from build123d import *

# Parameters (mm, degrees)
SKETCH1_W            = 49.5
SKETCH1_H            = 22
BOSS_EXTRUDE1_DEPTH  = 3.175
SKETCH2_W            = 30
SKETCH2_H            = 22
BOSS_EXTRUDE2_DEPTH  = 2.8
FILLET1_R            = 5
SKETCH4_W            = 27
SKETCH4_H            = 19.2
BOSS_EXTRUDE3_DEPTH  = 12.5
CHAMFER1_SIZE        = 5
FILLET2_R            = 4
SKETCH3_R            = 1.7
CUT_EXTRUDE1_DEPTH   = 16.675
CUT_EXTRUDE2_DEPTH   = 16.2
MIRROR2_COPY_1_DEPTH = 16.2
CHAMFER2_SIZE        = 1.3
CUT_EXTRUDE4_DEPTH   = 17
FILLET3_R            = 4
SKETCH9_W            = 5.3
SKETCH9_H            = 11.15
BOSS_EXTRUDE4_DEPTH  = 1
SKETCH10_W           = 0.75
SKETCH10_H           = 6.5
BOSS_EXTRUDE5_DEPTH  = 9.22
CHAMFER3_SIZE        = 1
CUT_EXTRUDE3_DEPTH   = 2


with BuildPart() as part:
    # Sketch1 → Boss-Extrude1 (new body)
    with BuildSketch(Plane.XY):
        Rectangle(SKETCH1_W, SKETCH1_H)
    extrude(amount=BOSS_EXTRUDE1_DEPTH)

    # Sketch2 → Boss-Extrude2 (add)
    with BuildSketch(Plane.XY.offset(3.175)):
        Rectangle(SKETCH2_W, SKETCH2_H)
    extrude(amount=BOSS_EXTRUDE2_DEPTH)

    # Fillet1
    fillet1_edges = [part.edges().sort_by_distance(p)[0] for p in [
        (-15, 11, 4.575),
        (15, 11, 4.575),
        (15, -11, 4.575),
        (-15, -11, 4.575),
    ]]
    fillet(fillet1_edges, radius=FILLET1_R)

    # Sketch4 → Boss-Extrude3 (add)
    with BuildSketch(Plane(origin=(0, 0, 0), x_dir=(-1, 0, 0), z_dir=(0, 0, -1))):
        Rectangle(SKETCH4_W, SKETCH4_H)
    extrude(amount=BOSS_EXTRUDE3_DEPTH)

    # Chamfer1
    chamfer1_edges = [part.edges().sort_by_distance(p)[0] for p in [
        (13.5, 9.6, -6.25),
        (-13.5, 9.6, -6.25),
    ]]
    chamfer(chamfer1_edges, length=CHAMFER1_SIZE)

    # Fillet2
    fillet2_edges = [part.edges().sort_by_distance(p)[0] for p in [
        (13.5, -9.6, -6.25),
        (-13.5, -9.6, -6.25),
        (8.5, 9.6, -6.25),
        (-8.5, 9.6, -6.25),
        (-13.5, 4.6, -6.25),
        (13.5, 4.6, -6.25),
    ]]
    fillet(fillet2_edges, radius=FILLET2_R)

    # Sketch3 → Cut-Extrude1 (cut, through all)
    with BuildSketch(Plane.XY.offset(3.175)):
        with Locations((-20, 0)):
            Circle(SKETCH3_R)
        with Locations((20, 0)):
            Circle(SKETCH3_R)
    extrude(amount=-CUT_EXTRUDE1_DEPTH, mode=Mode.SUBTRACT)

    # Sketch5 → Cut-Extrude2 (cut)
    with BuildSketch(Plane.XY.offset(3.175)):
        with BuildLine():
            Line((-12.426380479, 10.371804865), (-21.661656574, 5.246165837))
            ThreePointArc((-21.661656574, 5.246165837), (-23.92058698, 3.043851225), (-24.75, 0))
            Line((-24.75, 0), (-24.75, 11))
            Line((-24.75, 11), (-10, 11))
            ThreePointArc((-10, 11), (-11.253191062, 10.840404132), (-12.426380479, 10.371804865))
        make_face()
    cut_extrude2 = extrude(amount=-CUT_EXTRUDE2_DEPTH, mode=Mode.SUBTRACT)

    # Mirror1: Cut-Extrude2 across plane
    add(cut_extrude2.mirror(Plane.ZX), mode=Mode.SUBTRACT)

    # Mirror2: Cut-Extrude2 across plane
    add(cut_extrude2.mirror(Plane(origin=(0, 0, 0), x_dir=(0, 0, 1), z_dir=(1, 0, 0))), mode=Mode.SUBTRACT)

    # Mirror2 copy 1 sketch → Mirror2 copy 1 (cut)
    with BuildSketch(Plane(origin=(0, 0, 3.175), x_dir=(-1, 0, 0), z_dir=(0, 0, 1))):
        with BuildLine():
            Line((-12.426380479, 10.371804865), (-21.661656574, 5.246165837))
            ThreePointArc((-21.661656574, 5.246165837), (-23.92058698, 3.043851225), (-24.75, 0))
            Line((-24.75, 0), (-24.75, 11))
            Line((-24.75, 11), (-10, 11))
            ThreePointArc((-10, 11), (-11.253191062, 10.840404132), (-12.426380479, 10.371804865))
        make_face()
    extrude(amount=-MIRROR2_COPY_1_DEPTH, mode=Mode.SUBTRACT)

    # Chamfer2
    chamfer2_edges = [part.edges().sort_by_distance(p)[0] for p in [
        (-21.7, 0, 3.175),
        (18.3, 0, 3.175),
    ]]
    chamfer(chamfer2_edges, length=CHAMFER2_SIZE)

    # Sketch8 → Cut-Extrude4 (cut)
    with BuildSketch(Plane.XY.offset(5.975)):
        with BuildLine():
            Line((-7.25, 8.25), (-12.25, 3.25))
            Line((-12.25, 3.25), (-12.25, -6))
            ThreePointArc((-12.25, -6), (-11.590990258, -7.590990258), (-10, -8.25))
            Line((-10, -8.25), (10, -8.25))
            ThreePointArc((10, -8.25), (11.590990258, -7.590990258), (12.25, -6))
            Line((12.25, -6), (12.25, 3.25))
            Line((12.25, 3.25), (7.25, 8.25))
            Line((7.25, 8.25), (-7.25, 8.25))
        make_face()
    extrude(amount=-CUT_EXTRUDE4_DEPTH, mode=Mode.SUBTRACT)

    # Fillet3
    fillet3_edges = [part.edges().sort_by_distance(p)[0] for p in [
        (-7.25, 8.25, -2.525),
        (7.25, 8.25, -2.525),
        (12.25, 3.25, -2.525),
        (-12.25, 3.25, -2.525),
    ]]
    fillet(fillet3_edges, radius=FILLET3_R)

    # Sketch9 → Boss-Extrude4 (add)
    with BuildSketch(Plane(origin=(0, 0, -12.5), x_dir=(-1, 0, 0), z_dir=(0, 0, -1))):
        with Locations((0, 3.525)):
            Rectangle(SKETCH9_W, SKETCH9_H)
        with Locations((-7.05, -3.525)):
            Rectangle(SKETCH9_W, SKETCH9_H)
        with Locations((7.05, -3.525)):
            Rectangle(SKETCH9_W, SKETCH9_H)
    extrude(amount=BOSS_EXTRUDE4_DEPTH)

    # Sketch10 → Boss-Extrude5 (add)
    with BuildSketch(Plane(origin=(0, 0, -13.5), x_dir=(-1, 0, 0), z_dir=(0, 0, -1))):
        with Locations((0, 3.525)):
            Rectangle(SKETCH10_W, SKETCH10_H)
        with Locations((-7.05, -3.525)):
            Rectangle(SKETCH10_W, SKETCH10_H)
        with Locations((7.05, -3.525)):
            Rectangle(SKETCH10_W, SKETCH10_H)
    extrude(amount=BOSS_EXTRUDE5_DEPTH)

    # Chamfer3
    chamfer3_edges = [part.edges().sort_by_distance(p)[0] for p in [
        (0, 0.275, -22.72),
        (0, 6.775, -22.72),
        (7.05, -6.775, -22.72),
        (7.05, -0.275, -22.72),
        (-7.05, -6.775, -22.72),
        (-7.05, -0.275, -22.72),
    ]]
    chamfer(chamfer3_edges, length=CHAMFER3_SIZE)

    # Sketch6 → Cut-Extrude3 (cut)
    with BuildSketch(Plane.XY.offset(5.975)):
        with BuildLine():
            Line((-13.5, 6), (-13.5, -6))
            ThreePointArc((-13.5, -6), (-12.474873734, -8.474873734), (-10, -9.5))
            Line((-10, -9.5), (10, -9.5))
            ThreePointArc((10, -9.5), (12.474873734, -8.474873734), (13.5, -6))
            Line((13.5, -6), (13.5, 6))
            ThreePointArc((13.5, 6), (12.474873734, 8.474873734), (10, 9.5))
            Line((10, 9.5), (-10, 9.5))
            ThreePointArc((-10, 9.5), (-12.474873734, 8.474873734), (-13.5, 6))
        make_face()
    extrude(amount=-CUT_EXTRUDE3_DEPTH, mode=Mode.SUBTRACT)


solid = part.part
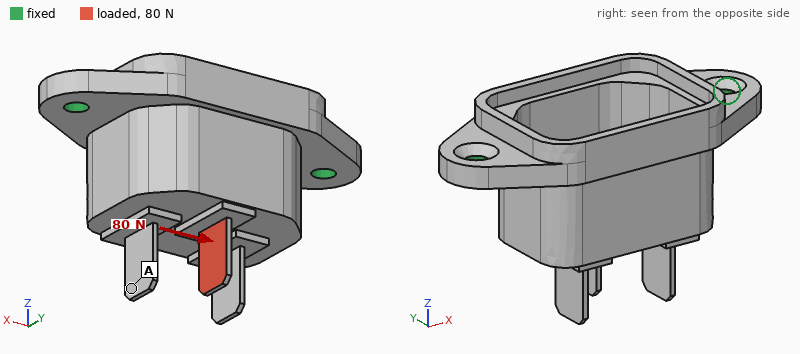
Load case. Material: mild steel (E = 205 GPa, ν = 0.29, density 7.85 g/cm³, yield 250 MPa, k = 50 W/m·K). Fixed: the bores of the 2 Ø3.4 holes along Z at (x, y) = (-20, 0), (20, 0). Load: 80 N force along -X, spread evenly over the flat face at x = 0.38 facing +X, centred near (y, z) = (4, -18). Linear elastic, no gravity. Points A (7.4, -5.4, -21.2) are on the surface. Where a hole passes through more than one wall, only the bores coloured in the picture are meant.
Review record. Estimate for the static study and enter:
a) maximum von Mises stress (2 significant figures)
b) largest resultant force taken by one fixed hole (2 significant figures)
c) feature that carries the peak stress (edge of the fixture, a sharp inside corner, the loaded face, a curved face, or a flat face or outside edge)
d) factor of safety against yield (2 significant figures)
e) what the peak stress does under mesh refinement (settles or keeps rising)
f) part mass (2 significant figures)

450 MPa
62 N
the loaded face
0.56
settles
33 g
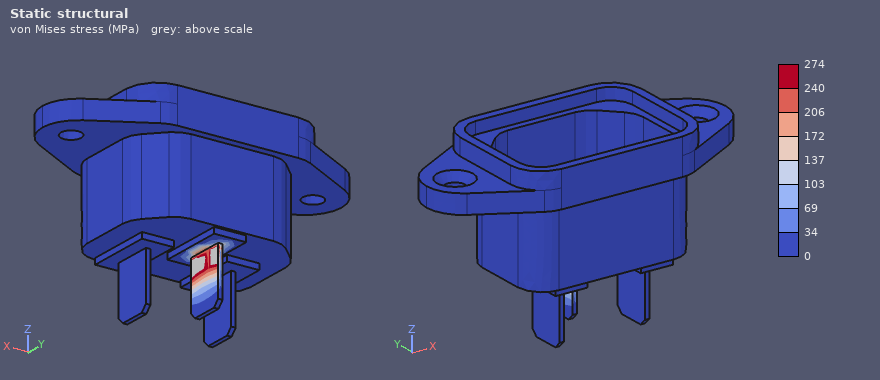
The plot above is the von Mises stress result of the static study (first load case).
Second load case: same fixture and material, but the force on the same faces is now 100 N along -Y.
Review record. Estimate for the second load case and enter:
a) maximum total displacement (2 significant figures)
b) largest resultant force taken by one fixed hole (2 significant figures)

27 µm
51 N
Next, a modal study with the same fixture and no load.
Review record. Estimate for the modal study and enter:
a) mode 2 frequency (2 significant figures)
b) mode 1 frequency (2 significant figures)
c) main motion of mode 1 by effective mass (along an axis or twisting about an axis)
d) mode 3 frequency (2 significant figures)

7200 Hz
4300 Hz
along Y
7300 Hz
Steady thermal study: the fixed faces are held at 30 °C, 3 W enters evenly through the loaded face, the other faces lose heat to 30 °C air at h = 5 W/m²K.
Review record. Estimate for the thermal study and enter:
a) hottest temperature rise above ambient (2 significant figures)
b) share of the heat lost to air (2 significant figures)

82 K
8.2 %
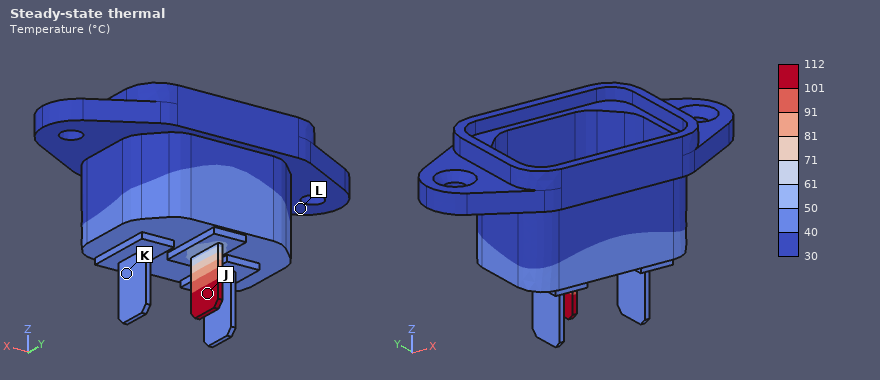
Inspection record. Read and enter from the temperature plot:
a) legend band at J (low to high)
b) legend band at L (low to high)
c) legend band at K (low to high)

101 to 112 °C
30 to 40 °C
40 to 50 °C
